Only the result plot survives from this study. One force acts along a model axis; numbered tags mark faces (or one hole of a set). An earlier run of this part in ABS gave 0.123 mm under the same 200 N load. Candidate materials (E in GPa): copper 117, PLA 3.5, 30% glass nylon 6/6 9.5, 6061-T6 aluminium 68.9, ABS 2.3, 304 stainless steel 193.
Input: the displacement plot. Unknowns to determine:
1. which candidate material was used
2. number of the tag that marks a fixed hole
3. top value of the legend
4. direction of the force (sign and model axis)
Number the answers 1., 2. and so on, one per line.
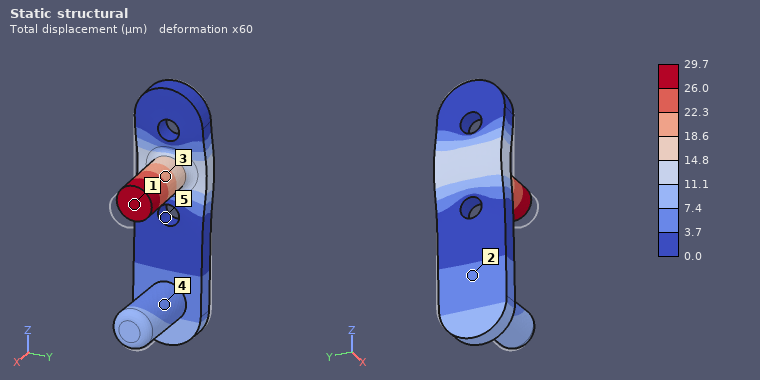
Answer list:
1. 30% glass nylon 6/6
2. 5
3. 29.7 µm
4. -X
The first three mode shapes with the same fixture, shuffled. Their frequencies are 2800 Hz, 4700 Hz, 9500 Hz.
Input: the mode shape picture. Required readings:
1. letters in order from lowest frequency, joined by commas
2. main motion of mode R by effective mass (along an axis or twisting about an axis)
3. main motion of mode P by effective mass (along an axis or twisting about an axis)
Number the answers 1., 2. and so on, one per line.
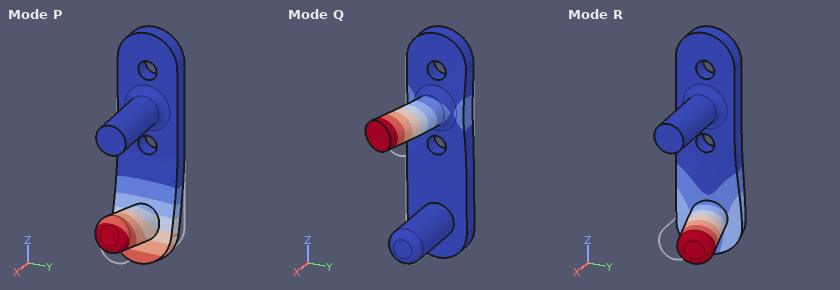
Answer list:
1. P, R, Q
2. along Y
3. along X
